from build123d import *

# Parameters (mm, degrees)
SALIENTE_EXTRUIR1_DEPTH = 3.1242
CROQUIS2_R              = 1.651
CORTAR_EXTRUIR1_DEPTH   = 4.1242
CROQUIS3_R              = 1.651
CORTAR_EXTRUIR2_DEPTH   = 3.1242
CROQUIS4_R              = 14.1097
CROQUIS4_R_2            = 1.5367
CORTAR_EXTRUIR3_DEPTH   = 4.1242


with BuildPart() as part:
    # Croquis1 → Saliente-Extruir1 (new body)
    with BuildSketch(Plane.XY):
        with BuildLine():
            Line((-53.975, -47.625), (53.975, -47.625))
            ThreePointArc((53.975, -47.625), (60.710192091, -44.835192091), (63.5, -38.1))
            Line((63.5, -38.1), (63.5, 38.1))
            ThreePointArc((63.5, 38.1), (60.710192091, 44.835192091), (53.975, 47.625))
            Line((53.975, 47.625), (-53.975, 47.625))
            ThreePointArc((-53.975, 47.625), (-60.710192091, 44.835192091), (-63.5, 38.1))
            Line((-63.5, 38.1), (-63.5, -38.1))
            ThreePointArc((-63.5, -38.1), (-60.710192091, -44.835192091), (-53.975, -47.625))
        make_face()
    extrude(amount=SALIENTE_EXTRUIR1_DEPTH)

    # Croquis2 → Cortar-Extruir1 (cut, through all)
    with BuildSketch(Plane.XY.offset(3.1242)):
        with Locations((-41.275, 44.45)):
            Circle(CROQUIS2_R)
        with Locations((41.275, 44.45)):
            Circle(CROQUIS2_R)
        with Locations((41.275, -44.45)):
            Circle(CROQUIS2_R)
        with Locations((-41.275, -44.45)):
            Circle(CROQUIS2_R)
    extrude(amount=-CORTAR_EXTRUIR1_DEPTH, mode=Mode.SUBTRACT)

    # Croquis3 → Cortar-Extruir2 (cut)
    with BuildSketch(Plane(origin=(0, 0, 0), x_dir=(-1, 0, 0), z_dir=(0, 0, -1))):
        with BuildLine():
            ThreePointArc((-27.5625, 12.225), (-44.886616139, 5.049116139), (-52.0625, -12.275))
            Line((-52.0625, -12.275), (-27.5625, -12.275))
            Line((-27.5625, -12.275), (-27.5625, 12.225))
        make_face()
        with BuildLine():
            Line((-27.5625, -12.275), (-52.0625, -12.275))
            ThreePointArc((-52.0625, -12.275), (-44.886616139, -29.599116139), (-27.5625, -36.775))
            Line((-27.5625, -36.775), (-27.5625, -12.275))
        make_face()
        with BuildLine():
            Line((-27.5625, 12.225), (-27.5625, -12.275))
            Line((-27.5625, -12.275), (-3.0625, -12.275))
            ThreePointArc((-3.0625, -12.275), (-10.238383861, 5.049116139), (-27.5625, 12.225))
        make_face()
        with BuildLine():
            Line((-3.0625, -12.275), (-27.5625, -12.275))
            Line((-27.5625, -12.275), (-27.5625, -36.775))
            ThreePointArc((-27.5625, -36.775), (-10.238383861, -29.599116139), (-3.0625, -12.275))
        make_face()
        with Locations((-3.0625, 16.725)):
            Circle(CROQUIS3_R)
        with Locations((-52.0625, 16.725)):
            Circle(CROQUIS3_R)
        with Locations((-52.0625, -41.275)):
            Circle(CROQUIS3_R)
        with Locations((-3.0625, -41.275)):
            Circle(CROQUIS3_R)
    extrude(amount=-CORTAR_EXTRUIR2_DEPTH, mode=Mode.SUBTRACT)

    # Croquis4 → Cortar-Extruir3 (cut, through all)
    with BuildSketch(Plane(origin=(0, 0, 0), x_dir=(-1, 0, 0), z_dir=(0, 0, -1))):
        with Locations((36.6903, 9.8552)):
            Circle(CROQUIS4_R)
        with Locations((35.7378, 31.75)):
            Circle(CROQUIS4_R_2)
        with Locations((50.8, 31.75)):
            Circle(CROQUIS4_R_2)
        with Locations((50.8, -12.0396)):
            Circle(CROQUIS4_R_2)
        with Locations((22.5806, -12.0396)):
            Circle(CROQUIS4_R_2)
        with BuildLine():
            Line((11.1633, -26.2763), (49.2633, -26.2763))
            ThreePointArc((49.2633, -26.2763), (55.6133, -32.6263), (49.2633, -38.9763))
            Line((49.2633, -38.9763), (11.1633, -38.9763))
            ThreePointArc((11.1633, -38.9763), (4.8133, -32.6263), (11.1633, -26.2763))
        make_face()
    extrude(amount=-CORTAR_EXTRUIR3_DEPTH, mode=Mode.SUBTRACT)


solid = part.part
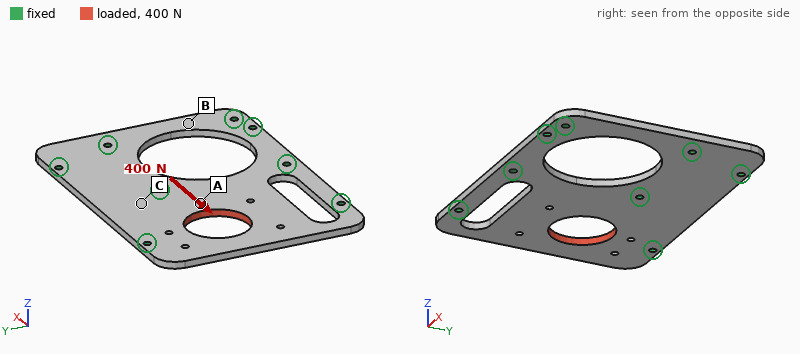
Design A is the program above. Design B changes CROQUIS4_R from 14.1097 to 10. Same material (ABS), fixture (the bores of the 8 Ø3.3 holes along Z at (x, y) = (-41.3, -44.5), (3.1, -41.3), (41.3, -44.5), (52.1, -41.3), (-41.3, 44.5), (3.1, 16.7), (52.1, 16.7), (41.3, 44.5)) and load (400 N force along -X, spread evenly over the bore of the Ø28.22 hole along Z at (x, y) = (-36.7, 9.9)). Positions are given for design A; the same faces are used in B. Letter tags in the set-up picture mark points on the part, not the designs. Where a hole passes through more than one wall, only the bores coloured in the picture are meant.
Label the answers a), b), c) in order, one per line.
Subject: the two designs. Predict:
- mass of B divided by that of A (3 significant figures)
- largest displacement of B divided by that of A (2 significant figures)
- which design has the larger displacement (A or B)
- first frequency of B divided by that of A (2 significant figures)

a) 1.04
b) 0.81
c) A
d) 0.99
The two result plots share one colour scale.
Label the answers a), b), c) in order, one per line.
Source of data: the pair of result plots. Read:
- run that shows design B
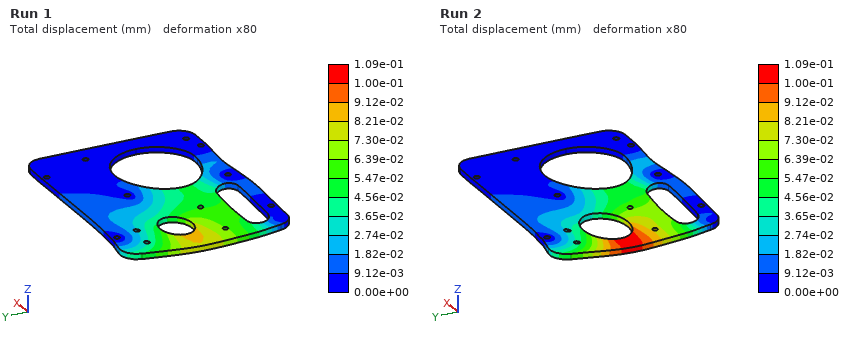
a) Run 1
